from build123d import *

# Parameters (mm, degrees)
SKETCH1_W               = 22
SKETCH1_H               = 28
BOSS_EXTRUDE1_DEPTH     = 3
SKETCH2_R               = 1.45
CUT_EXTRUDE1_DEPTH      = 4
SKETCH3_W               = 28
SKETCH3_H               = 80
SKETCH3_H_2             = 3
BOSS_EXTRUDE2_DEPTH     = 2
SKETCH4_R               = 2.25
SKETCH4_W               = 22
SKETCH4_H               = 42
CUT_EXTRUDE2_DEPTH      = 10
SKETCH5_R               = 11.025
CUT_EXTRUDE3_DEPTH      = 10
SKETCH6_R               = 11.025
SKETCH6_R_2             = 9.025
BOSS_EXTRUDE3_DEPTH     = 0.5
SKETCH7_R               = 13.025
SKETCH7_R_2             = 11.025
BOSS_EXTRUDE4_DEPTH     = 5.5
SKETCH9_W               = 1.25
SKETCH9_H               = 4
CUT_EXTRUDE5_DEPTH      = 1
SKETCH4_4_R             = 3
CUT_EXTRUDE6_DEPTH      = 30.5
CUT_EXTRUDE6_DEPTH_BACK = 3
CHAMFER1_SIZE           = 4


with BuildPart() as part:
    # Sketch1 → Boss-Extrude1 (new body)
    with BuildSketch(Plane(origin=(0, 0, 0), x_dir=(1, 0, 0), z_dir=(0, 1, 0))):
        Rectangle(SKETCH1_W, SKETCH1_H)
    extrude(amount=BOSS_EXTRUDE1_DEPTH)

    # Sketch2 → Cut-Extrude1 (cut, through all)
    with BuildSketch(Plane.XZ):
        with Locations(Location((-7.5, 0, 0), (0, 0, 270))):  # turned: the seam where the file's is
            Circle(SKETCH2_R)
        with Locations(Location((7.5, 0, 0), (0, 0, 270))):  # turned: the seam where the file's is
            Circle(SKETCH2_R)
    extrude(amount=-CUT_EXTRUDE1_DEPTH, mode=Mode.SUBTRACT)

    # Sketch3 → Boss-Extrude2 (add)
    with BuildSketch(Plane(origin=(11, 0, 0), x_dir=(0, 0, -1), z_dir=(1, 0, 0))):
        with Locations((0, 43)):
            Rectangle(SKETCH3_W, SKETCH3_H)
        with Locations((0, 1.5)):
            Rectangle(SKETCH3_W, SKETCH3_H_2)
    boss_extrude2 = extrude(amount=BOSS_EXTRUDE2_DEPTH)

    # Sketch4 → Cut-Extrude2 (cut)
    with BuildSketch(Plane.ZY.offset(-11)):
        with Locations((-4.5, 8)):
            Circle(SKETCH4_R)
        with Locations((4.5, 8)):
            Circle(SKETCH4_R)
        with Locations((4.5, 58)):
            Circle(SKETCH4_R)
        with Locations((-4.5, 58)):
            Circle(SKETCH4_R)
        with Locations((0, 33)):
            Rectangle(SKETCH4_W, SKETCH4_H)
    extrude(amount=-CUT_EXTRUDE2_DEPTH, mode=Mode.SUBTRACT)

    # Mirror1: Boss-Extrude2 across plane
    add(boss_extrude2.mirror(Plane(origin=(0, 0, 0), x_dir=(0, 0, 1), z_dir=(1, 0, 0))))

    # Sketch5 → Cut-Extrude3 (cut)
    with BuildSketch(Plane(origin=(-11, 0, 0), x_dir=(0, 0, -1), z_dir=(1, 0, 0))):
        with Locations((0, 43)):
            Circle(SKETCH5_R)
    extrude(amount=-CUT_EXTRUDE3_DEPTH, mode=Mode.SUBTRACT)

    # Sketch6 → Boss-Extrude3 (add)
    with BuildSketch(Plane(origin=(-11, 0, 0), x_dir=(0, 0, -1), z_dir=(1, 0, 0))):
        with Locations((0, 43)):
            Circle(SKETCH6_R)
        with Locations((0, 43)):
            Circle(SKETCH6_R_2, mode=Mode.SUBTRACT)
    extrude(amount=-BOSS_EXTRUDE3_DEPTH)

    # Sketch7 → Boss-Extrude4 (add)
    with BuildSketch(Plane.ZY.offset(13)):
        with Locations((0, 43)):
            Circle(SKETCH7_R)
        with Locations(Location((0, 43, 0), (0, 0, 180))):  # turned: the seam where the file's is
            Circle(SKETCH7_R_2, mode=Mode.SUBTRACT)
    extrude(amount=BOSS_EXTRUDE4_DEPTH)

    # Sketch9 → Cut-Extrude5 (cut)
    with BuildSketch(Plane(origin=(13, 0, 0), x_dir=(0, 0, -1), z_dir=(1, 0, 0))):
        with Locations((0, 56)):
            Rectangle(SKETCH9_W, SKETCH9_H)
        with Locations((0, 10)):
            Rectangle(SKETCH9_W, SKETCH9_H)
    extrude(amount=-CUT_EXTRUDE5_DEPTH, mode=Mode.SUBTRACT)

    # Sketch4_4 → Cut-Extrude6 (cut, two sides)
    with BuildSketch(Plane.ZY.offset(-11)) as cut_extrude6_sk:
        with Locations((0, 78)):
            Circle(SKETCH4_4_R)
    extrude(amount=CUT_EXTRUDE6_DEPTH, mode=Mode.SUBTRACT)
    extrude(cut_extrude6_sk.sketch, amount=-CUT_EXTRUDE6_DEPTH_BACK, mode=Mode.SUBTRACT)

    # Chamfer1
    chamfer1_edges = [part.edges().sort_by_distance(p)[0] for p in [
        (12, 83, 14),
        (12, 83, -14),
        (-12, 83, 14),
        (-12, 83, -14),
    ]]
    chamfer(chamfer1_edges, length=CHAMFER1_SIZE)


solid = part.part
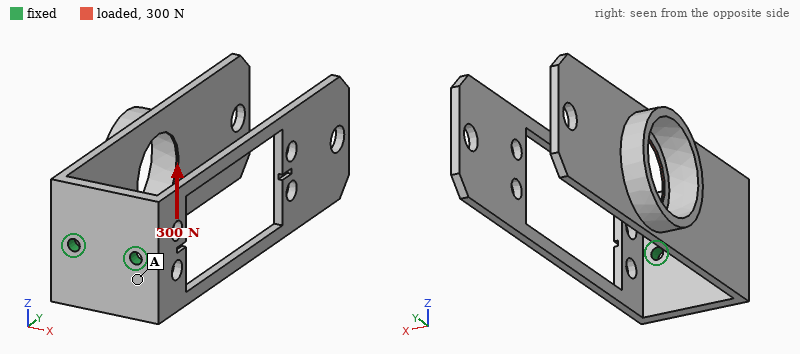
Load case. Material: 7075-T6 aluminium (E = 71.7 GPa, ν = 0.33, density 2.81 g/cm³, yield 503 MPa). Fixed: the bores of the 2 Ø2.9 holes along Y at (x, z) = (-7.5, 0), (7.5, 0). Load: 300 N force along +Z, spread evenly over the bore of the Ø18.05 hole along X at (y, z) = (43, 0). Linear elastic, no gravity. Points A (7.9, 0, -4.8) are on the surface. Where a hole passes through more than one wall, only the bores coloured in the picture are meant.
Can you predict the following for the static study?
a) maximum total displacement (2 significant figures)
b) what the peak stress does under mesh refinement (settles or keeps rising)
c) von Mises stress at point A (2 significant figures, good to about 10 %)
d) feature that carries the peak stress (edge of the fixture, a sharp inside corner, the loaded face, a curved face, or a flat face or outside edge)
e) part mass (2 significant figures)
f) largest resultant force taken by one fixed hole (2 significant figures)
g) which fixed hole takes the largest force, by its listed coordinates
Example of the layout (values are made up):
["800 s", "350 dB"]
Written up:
["1.0 mm", "keeps rising", "42 MPa", "edge of the fixture", "25 g", "350 N", "(-7.5, 0)"]
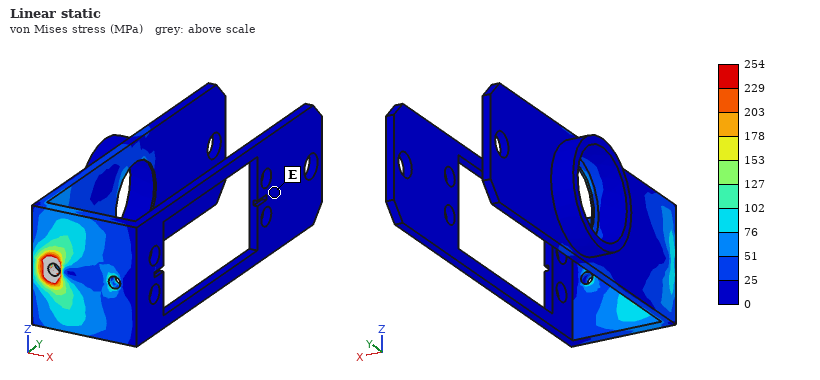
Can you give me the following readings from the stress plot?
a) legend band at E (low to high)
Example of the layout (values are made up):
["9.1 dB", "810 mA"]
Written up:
["0 to 25 MPa"]
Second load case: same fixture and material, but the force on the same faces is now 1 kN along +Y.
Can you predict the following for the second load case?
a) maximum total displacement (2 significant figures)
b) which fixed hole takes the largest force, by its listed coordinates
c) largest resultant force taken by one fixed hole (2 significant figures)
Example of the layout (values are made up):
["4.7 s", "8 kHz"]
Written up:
["1.00 mm", "(-7.5, 0)", "1.1 kN"]
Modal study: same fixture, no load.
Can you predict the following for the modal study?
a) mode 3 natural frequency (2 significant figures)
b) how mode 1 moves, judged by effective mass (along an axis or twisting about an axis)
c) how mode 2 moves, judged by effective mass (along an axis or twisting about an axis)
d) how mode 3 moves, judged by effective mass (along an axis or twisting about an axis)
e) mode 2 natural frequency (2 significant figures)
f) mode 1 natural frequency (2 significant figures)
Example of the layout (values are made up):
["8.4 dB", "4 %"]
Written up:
["560 Hz", "along X", "along X", "along Z", "260 Hz", "150 Hz"]
